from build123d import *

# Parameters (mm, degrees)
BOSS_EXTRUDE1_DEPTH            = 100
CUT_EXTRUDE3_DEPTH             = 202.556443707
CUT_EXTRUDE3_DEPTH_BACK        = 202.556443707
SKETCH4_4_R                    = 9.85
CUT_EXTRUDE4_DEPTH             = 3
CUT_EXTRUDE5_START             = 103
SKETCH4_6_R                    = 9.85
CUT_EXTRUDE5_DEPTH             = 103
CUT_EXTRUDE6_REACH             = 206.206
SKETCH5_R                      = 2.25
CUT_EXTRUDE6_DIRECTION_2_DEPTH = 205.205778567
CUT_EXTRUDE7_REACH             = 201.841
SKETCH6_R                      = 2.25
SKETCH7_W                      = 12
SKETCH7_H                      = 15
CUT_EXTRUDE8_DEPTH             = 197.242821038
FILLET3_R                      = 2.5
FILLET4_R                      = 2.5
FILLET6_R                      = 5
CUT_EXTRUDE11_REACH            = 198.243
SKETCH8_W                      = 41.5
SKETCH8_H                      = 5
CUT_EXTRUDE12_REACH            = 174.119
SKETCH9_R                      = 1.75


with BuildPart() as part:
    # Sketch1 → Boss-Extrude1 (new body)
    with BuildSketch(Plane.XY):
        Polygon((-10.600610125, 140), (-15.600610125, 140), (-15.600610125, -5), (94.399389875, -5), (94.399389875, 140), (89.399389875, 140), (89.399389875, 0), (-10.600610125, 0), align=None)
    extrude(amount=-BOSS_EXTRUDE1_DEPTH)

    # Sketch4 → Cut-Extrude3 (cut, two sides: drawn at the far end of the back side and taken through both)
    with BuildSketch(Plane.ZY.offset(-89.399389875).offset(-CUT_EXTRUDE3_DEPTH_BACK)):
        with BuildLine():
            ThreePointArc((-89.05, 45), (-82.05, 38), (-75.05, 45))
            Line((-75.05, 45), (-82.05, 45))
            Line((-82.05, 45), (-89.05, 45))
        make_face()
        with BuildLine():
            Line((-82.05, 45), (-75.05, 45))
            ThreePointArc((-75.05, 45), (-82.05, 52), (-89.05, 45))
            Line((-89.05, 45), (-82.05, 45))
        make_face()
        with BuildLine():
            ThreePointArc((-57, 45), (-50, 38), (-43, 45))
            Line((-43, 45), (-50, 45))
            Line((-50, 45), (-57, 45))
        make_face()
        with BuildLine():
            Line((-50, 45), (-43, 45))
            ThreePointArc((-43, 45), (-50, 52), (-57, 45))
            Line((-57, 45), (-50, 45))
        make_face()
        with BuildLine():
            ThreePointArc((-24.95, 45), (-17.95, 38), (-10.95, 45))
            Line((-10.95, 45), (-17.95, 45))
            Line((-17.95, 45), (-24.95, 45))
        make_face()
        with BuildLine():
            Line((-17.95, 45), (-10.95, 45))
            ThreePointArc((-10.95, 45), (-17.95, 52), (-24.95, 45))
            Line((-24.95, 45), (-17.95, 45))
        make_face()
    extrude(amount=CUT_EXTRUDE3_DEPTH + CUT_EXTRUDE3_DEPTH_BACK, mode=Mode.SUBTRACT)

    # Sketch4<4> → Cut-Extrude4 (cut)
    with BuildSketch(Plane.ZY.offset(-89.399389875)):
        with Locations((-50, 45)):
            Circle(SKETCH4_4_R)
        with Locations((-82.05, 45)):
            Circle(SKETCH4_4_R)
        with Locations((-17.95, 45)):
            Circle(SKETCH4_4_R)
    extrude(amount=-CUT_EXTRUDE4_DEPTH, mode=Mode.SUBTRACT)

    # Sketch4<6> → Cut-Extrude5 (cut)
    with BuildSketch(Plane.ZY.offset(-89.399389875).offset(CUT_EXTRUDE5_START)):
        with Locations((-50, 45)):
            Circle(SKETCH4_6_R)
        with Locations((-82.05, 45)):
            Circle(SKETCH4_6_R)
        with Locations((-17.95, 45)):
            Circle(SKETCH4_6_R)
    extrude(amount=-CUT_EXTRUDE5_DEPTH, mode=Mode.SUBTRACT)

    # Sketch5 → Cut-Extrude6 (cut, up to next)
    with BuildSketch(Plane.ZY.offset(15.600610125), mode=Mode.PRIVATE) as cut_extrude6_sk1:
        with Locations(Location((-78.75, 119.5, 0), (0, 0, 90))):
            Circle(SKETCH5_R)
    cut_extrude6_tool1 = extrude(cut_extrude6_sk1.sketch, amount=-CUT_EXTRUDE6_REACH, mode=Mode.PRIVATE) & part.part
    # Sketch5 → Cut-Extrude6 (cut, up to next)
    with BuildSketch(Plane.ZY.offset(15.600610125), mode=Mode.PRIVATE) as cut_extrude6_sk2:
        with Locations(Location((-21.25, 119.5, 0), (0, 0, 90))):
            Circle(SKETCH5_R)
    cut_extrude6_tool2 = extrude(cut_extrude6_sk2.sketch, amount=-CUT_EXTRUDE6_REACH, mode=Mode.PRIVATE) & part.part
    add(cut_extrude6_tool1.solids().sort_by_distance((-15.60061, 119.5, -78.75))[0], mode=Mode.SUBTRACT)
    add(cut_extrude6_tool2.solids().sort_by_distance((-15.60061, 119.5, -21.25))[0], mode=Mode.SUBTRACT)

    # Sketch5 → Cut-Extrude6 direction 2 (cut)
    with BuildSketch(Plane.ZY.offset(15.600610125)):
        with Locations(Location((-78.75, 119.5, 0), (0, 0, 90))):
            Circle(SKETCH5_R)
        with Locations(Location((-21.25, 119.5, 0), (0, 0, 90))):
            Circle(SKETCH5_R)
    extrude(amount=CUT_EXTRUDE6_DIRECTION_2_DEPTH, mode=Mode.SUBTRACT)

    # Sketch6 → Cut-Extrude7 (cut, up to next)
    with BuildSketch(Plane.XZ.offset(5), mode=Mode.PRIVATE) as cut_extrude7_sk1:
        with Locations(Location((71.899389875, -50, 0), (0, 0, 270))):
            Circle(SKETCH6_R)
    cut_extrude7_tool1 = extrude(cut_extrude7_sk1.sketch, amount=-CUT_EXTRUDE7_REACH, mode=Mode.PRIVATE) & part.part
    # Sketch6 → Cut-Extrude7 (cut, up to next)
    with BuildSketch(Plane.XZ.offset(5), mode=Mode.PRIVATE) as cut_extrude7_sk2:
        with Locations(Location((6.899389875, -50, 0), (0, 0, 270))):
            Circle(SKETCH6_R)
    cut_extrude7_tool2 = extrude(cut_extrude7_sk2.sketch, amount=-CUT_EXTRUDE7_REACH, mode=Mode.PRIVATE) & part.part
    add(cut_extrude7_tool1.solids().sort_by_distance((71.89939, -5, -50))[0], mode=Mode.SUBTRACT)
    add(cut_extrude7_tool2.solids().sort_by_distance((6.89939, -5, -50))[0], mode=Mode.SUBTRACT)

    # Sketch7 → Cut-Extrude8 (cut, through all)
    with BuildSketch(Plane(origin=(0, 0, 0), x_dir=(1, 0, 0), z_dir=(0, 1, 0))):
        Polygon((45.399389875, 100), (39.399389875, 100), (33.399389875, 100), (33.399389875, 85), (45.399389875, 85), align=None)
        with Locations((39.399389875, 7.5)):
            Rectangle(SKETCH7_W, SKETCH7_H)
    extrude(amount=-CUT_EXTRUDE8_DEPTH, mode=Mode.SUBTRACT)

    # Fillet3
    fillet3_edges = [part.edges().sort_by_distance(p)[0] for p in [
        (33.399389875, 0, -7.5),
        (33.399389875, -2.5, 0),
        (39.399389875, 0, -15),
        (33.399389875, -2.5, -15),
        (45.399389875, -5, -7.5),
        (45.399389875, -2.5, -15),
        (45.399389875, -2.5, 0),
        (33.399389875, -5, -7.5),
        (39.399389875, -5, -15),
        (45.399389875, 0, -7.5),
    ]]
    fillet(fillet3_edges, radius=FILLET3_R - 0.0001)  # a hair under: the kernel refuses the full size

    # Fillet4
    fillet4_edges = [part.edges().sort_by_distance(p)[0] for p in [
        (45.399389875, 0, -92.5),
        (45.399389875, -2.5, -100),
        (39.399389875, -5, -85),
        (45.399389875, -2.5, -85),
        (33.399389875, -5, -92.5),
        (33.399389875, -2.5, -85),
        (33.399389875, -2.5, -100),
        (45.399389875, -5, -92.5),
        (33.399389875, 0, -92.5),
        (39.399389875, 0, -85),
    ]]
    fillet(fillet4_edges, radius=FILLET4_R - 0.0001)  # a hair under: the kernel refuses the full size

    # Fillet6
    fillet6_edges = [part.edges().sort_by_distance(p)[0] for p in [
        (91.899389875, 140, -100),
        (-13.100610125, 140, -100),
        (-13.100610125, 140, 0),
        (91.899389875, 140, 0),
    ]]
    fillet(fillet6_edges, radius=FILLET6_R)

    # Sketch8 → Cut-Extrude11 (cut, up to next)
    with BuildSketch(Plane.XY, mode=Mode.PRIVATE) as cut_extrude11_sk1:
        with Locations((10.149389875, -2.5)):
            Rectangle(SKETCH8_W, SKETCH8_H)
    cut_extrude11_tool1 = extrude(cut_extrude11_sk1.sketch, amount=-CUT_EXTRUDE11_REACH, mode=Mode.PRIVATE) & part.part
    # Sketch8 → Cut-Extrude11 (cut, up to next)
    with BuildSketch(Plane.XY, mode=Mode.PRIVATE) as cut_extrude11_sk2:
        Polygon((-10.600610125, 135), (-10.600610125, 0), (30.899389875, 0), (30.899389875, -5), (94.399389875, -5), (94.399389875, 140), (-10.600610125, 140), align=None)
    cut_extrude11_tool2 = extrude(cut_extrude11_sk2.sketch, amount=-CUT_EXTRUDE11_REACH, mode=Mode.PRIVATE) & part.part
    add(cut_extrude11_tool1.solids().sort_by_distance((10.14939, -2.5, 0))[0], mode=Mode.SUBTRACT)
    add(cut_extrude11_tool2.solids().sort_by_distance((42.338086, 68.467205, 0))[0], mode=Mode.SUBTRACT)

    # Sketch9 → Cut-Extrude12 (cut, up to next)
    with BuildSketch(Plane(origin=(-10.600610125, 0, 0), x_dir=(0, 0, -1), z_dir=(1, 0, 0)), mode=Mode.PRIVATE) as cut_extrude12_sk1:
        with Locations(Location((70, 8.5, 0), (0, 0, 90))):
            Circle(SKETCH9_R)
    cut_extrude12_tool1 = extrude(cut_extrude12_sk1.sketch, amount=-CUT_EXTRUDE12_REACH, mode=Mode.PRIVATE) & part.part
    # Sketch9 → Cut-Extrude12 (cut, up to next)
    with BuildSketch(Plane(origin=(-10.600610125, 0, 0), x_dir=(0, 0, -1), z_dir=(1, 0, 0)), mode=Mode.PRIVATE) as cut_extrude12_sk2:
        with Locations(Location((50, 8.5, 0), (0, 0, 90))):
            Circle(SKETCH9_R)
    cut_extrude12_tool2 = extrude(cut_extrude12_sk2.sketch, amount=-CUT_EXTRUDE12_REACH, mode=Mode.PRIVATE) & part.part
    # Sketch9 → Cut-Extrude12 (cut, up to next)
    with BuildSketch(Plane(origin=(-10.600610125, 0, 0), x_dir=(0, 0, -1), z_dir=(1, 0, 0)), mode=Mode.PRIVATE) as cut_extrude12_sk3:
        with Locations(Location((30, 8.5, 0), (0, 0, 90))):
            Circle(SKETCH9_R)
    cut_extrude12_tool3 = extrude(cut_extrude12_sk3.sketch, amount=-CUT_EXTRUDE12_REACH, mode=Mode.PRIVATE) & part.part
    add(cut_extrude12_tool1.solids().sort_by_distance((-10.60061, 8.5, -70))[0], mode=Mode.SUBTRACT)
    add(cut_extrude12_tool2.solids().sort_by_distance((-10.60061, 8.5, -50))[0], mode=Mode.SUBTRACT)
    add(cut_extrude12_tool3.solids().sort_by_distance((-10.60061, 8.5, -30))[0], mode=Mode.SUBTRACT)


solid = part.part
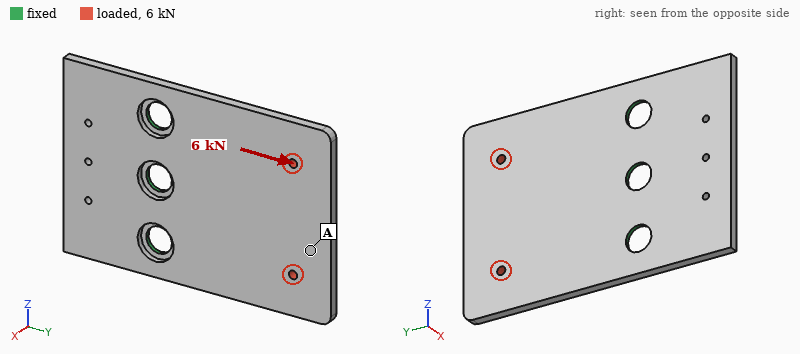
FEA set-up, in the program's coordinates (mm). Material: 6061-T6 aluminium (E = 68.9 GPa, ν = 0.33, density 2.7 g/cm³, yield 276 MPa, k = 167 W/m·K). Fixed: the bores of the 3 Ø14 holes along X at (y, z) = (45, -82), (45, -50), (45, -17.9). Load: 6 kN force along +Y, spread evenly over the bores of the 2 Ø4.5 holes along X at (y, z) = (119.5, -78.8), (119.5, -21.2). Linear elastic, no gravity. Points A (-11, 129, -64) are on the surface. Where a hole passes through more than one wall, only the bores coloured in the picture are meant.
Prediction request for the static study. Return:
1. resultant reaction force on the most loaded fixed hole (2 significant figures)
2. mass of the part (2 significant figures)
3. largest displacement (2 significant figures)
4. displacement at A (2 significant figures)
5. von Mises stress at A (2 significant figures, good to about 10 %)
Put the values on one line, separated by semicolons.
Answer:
2.1 kN; 180 g; 0.14 mm; 0.12 mm; 8.5 MPa
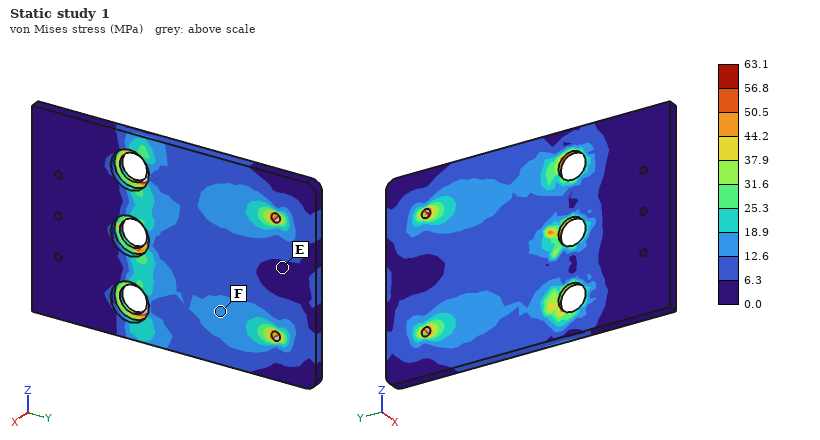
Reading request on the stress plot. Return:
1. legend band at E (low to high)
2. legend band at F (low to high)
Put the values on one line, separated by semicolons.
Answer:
0.0 to 6.3 MPa; 12.6 to 18.9 MPa
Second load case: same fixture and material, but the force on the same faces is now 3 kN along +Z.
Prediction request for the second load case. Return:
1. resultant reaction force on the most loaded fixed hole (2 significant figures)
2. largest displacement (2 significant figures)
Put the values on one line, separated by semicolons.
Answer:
3.2 kN; 74 µm
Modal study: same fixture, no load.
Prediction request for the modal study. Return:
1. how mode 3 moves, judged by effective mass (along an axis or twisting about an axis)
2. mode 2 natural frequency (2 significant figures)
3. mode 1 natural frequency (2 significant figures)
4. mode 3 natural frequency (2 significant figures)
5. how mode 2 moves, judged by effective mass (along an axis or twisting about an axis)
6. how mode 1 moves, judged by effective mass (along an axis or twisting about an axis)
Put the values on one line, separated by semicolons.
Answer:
along X; 1000 Hz; 430 Hz; 1500 Hz; twisting about Y; along X
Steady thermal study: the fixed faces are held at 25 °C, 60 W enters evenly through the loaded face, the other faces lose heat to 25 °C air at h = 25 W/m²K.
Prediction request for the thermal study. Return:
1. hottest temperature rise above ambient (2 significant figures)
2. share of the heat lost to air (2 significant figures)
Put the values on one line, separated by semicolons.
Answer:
54 K; 24 %
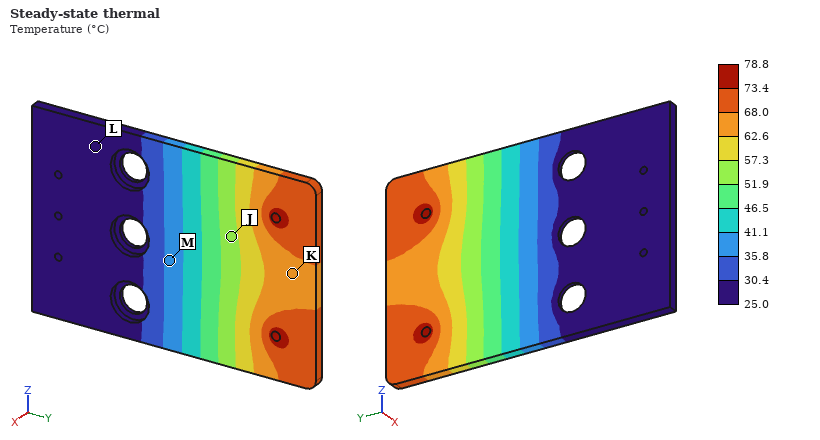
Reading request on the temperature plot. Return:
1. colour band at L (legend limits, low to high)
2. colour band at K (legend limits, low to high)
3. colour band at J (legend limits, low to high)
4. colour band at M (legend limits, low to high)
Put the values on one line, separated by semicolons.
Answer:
25.0 to 30.4 °C; 62.6 to 68.0 °C; 51.9 to 57.3 °C; 35.8 to 41.1 °C
